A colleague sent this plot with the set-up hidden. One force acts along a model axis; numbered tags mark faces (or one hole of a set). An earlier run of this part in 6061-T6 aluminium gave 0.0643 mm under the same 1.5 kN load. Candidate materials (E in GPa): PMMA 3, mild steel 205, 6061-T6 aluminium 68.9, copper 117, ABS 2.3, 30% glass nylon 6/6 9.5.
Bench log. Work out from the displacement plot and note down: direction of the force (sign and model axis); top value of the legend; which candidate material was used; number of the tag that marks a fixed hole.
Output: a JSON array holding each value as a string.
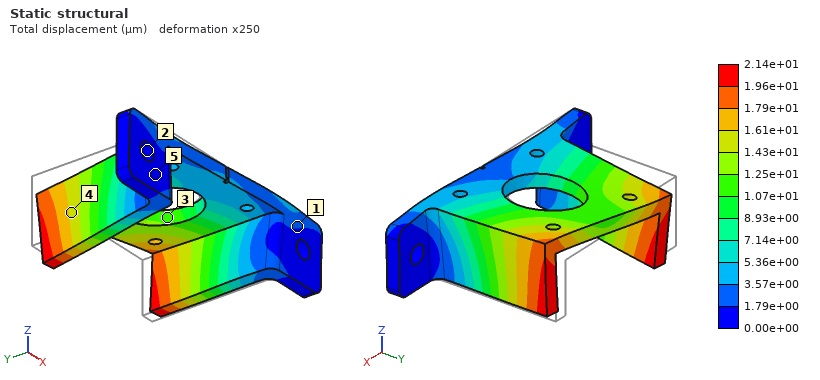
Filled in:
["+X", "2.14e+01 µm", "mild steel", "2"]
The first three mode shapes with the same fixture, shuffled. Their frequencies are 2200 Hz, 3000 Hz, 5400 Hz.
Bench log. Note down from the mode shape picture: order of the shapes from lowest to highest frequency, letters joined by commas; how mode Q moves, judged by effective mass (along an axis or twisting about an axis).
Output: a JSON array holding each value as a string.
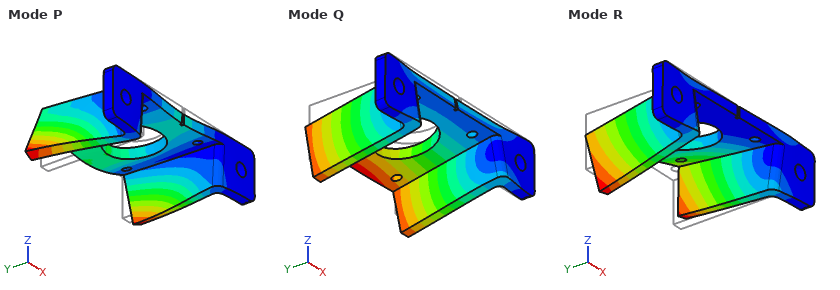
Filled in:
["Q, R, P", "along Z"]
